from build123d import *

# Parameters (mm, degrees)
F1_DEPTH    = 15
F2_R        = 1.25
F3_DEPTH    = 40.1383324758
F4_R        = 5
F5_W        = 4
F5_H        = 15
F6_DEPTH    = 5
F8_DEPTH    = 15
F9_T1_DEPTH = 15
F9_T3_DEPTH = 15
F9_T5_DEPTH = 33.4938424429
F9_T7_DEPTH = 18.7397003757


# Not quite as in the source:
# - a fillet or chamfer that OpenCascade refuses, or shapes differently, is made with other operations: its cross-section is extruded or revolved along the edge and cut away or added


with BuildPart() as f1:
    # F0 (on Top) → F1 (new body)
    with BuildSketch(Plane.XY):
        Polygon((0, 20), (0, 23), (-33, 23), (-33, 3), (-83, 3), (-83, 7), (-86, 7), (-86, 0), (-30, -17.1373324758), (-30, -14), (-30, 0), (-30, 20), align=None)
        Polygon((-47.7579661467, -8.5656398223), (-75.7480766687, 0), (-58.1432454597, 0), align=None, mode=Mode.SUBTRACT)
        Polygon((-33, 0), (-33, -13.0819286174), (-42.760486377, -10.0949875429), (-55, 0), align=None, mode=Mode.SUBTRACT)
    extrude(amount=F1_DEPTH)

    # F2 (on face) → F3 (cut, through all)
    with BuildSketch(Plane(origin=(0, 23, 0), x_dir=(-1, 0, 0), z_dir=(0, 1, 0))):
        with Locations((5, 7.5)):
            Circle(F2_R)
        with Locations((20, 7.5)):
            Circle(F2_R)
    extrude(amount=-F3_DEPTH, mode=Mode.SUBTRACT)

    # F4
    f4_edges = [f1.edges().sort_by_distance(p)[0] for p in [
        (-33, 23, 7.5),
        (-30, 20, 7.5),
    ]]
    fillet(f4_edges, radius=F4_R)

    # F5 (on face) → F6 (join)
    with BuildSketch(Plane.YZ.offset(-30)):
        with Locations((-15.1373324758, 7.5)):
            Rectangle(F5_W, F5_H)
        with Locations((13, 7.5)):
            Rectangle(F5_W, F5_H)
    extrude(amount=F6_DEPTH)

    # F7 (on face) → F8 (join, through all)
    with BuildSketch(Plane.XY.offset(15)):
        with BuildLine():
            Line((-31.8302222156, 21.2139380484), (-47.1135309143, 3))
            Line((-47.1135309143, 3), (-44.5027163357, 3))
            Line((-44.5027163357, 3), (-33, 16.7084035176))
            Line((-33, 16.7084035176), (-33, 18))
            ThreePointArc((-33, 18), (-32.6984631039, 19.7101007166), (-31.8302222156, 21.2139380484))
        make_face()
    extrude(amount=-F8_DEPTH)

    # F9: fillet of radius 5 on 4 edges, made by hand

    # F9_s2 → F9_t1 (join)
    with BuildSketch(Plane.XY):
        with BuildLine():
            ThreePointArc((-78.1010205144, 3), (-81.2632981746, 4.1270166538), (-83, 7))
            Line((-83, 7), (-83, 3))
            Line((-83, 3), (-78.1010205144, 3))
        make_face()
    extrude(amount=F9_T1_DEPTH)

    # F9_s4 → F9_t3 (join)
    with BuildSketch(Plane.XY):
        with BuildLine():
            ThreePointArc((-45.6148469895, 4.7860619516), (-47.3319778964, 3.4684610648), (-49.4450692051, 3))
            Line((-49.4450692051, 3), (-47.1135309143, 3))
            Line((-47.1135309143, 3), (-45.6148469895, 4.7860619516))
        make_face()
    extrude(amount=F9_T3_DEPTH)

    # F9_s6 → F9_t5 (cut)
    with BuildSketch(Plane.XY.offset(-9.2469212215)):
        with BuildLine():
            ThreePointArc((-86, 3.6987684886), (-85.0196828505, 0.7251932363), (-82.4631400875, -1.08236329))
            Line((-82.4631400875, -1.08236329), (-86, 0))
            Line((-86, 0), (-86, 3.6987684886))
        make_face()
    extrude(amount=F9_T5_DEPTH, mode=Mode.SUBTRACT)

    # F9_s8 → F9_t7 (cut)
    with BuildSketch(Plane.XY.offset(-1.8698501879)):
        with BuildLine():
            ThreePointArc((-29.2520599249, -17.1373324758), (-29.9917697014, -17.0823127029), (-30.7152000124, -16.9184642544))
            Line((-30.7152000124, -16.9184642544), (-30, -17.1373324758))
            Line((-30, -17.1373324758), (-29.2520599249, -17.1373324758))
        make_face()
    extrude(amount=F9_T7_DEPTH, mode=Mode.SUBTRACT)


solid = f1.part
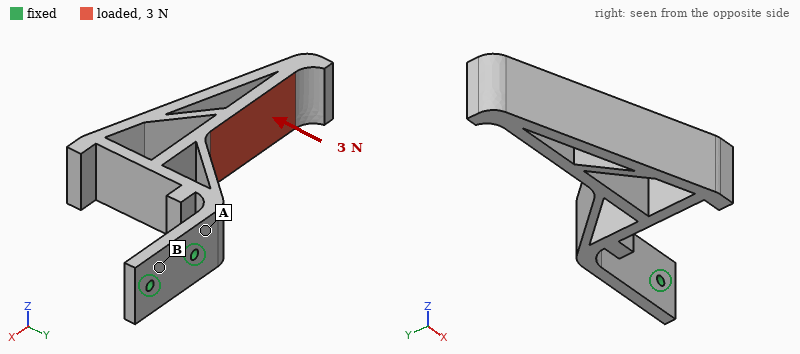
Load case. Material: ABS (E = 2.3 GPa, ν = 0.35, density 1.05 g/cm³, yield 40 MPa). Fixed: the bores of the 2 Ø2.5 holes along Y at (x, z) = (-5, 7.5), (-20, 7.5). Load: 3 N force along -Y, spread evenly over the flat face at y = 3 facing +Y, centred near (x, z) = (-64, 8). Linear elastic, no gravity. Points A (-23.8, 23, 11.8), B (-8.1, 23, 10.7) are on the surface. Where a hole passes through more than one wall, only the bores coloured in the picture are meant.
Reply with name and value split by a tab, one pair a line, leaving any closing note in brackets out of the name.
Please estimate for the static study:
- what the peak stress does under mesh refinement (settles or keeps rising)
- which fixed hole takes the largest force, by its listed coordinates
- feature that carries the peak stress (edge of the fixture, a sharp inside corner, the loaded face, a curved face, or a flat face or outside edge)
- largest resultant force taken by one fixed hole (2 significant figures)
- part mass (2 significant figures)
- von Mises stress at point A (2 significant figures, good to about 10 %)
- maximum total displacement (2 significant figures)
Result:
what the peak stress does under mesh refinement	keeps rising
which fixed hole takes the largest force, by its listed coordinates	(-20, 7.5)
feature that carries the peak stress	edge of the fixture
largest resultant force taken by one fixed hole	5.6 N
part mass	10 g
von Mises stress at point A	4.6 MPa
maximum total displacement	1.1 mm
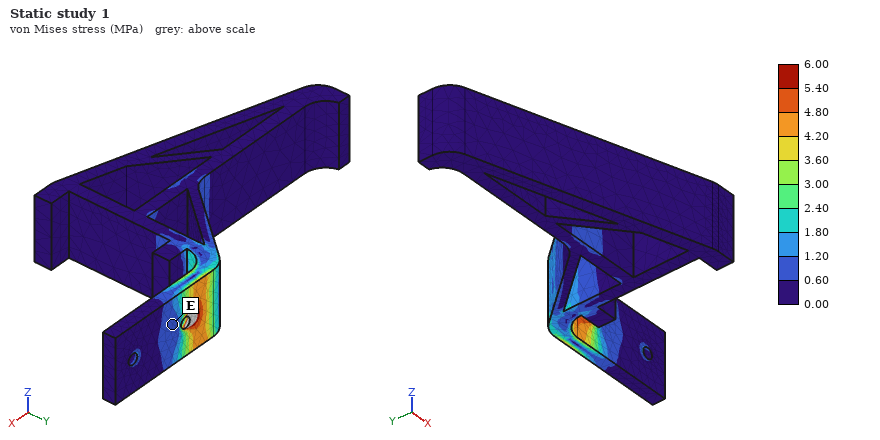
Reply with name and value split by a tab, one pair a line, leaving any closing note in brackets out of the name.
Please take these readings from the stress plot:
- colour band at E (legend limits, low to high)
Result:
colour band at E	0.60 to 1.20 MPa
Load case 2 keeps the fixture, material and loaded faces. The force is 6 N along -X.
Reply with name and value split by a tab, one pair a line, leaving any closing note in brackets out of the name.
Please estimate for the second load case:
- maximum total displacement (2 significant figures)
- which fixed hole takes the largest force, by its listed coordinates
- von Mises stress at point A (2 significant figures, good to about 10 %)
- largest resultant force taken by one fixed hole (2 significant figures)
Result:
maximum total displacement	0.97 mm
which fixed hole takes the largest force, by its listed coordinates	(-20, 7.5)
von Mises stress at point A	4.2 MPa
largest resultant force taken by one fixed hole	5.6 N
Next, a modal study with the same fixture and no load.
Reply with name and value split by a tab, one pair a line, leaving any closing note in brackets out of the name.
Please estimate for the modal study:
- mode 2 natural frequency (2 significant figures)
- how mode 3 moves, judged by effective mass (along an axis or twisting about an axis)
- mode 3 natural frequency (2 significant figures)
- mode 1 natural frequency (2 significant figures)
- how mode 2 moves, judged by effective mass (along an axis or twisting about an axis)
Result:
mode 2 natural frequency	250 Hz
how mode 3 moves, judged by effective mass	twisting about Y
mode 3 natural frequency	510 Hz
mode 1 natural frequency	120 Hz
how mode 2 moves, judged by effective mass	along Z
